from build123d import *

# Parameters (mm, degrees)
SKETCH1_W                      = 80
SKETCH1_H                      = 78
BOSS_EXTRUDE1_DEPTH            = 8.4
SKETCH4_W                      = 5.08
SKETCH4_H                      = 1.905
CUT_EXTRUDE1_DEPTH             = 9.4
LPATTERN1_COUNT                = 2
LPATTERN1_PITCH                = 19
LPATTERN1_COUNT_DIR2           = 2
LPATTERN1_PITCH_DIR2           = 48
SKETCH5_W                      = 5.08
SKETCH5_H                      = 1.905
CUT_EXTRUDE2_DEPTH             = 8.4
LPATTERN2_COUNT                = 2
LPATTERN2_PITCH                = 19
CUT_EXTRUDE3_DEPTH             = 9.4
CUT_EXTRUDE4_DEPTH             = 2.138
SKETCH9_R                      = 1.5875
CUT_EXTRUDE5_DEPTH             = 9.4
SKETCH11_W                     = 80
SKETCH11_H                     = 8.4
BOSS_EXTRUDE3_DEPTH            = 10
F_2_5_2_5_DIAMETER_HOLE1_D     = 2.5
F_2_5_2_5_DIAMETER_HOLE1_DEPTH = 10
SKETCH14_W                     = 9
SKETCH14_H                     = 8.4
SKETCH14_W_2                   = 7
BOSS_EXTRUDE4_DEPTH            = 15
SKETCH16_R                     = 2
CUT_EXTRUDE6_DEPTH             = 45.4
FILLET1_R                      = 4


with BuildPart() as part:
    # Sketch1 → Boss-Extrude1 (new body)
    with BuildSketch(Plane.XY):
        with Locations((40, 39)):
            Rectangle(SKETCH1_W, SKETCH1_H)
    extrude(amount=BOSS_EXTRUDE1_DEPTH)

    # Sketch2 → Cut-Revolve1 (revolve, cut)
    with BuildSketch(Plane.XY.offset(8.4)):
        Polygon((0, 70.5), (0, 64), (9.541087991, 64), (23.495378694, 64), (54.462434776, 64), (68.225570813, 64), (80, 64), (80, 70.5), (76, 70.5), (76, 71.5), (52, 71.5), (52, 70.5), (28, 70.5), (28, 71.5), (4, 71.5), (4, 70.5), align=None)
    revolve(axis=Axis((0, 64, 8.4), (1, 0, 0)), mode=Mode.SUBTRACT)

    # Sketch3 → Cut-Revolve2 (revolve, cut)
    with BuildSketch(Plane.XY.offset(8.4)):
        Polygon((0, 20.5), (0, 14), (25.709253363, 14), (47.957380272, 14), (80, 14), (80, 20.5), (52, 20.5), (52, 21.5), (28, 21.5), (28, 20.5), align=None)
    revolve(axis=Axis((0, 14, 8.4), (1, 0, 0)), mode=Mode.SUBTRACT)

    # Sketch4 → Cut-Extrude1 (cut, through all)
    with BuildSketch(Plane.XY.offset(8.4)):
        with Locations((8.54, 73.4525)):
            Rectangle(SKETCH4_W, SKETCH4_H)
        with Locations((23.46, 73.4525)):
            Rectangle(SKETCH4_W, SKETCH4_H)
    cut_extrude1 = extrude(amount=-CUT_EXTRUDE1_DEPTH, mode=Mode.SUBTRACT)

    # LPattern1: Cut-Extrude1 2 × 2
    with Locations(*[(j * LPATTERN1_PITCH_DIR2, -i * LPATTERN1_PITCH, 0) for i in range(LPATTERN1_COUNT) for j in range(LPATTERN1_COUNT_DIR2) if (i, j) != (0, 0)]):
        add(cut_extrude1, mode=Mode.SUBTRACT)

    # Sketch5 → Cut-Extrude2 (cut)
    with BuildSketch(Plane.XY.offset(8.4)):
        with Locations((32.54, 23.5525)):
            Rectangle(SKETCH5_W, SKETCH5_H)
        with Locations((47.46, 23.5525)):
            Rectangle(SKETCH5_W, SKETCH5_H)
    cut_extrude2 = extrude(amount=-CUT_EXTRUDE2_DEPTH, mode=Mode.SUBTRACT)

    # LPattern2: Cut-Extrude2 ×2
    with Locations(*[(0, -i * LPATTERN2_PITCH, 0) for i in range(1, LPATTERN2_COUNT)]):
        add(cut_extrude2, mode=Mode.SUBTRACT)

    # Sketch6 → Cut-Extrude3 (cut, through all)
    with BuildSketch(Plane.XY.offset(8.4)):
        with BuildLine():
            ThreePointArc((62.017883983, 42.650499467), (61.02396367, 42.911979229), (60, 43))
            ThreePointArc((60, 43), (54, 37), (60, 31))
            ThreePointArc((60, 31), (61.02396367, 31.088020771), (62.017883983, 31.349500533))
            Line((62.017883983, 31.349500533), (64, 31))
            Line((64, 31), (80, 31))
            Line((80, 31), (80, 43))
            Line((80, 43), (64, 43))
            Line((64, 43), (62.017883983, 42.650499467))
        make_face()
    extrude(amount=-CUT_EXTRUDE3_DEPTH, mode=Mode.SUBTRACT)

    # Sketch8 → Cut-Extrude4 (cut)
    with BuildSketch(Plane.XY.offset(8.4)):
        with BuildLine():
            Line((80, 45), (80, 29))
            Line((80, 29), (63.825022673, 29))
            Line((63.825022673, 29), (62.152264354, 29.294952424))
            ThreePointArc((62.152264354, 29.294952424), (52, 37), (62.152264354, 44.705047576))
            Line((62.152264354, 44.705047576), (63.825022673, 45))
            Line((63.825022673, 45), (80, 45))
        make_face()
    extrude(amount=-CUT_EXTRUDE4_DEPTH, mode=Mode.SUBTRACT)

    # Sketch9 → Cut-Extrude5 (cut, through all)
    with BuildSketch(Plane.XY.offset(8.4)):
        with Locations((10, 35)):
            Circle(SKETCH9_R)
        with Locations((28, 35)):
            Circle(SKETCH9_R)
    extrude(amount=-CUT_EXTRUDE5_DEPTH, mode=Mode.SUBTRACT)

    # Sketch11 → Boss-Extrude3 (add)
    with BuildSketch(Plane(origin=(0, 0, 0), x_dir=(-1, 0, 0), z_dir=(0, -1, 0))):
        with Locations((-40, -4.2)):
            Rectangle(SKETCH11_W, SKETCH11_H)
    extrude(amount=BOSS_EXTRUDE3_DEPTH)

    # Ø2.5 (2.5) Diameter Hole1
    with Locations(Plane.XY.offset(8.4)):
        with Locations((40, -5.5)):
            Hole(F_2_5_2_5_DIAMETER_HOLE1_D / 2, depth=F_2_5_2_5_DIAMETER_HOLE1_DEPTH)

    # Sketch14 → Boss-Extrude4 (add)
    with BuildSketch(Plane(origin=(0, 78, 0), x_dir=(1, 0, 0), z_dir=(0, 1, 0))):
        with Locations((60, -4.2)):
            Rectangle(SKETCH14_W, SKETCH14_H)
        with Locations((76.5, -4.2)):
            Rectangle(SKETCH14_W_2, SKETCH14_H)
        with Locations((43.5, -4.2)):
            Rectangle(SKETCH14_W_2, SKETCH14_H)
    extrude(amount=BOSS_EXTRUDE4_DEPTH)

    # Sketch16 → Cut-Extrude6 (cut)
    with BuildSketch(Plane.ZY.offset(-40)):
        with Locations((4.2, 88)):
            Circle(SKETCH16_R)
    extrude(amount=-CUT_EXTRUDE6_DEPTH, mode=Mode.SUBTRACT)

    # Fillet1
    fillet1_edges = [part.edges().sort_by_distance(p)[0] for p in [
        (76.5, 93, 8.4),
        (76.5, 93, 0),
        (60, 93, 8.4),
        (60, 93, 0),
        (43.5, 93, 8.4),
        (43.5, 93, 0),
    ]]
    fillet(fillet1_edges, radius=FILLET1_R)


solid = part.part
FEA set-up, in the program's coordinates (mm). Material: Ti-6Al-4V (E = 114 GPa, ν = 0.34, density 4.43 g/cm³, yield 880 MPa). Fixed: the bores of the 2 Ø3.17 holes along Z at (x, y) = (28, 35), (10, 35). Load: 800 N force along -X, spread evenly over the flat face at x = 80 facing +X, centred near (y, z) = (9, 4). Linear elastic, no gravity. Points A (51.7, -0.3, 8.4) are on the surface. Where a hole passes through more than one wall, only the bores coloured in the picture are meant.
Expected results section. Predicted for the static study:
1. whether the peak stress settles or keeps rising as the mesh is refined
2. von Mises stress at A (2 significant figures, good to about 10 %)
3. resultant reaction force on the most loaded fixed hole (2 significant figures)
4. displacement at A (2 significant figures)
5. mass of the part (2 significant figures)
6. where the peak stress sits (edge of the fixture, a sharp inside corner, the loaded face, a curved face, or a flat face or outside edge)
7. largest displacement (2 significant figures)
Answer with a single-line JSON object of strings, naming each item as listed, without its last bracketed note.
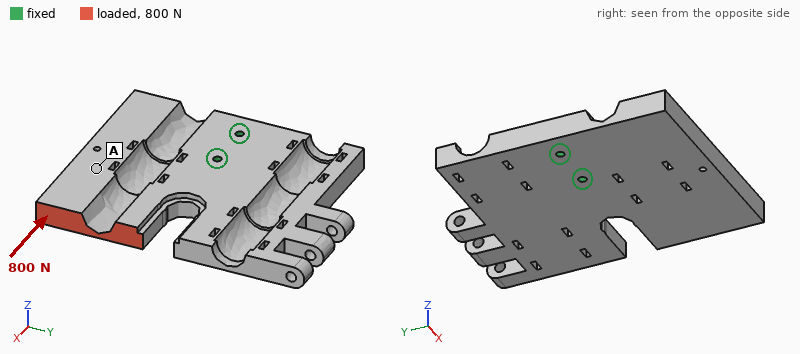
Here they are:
{"whether the peak stress settles or keeps rising as the mesh is refined": "keeps rising", "von Mises stress at A": "2.8 MPa", "resultant reaction force on the most loaded fixed hole": "1.2 kN", "displacement at A": "10 µm", "mass of the part": "200 g", "where the peak stress sits": "edge of the fixture", "largest displacement": "16 µm"}
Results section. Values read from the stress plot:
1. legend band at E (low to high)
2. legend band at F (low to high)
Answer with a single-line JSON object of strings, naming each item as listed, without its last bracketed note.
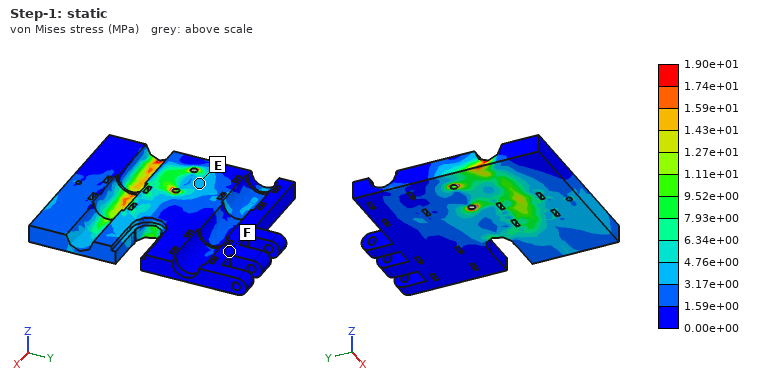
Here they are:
{"legend band at E": "3.17e+00 to 4.76e+00 MPa", "legend band at F": "0.00e+00 to 1.59e+00 MPa"}
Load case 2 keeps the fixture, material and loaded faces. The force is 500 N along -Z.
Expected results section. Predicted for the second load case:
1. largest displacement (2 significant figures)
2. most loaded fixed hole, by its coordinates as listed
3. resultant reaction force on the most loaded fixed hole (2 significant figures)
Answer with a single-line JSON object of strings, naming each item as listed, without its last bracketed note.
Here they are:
{"largest displacement": "0.36 mm", "most loaded fixed hole, by its coordinates as listed": "(28, 35)", "resultant reaction force on the most loaded fixed hole": "1.3 kN"}
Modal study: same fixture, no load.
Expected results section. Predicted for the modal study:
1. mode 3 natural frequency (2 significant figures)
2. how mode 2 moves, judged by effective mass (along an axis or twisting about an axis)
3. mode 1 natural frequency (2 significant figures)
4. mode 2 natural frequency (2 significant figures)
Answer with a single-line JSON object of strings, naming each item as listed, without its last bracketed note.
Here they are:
{"mode 3 natural frequency": "2100 Hz", "how mode 2 moves, judged by effective mass": "along Z", "mode 1 natural frequency": "990 Hz", "mode 2 natural frequency": "1100 Hz"}
